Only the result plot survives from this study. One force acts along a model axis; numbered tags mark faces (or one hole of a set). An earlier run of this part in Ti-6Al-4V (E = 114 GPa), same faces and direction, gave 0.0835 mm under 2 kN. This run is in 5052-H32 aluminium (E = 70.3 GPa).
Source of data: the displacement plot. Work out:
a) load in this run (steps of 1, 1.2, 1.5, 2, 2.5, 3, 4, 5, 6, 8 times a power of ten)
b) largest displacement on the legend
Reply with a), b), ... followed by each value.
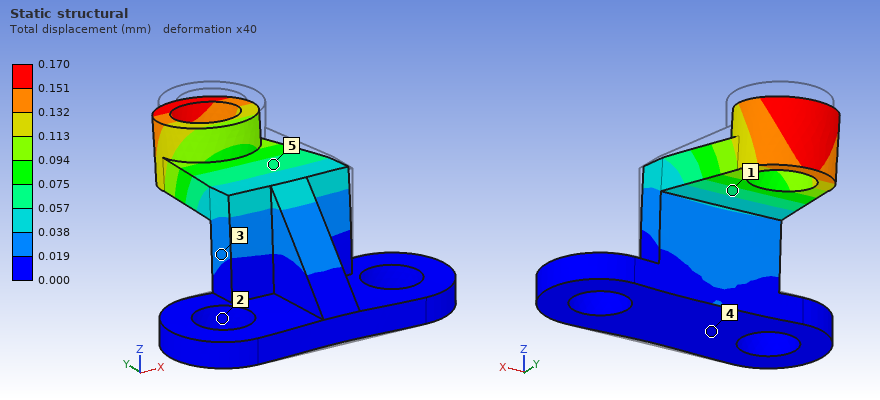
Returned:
a) 2.5 kN
b) 0.170 mm
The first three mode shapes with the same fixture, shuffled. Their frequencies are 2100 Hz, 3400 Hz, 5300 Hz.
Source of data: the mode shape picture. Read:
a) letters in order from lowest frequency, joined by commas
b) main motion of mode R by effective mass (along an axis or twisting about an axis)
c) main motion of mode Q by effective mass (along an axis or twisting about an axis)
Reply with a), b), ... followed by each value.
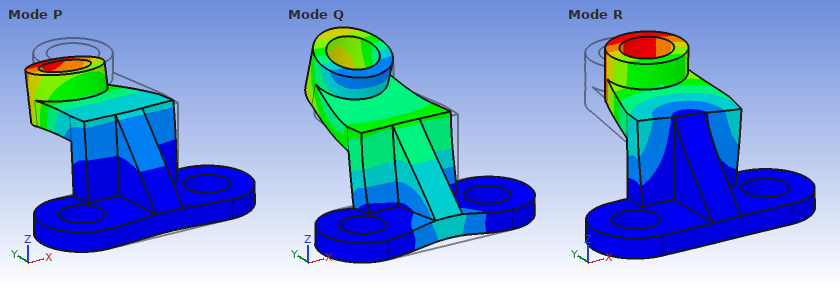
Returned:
a) P, R, Q
b) along X
c) along Y
